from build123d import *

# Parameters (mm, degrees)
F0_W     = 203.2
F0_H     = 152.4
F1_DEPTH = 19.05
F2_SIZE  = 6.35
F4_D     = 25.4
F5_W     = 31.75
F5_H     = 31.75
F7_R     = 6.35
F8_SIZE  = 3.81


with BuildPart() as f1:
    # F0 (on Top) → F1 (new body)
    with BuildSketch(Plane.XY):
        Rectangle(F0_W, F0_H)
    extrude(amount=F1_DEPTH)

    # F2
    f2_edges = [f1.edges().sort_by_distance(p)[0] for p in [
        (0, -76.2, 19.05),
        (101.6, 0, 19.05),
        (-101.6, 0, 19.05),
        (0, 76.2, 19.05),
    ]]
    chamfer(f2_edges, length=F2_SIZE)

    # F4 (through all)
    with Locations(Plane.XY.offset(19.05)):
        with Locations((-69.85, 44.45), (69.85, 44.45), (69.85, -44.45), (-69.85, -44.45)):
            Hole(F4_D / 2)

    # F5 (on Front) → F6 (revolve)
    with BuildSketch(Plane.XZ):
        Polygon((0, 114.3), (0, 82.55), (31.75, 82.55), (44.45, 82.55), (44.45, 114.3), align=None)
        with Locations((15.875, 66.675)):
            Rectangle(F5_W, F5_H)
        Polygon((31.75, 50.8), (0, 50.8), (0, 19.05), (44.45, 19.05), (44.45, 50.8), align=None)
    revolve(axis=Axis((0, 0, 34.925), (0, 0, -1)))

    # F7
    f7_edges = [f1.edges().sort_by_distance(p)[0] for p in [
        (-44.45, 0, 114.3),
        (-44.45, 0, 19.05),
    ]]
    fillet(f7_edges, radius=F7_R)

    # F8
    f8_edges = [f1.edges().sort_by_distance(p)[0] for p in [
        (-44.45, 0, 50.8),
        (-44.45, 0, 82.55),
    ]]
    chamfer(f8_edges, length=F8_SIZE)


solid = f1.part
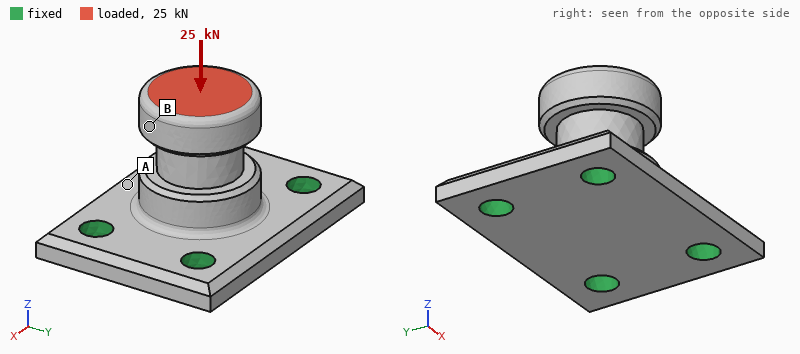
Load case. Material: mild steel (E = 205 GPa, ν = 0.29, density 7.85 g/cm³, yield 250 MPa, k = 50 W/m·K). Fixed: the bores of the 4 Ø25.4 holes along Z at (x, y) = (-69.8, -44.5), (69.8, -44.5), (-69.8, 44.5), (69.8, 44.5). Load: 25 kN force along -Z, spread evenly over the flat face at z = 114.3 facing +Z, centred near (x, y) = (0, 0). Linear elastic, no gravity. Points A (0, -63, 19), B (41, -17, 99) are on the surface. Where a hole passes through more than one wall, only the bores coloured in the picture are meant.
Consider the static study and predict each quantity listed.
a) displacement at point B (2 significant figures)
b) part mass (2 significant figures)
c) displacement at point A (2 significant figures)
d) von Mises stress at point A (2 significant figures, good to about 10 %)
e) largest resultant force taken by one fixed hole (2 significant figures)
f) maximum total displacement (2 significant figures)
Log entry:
9.9 µm
8.1 kg
6.3 µm
9.3 MPa
6.8 kN
10 µm
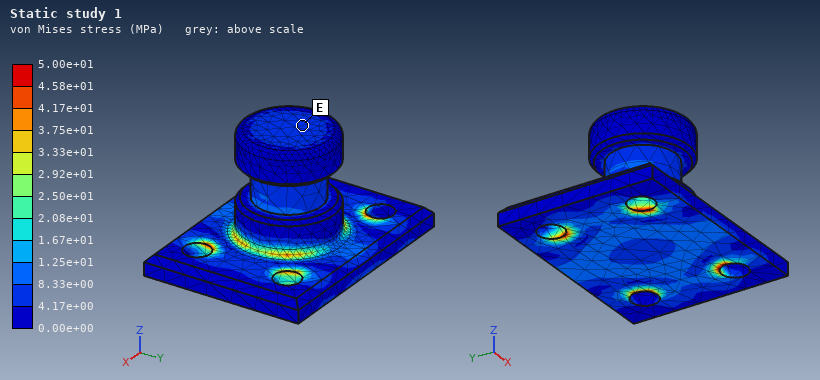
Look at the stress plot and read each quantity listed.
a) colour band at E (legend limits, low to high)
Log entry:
4.17e+00 to 8.33e+00 MPa
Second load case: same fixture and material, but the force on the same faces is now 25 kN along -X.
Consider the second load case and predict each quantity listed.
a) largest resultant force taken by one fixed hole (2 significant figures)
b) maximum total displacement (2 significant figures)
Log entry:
14 kN
68 µm
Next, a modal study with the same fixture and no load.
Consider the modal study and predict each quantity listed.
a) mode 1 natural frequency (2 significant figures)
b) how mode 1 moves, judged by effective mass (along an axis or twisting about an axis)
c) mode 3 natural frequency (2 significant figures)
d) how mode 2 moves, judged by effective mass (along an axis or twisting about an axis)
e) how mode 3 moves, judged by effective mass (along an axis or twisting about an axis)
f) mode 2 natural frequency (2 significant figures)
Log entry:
2200 Hz
along Y
3800 Hz
along X
along Z
2800 Hz
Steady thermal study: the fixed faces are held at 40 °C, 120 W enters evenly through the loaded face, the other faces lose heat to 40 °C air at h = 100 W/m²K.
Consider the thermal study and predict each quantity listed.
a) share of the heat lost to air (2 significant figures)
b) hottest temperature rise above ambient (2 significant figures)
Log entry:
68 %
44 K
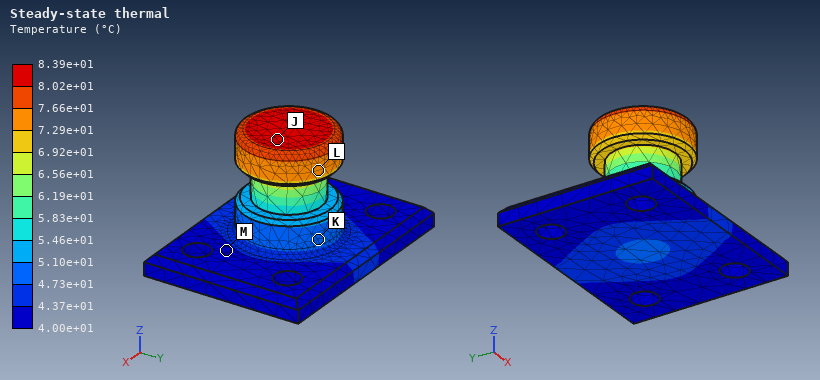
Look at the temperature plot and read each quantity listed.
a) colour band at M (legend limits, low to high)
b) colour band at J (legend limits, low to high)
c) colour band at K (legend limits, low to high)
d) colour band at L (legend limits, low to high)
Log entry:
4.00e+01 to 4.37e+01 °C
8.02e+01 to 8.39e+01 °C
4.73e+01 to 5.10e+01 °C
7.29e+01 to 7.66e+01 °C
